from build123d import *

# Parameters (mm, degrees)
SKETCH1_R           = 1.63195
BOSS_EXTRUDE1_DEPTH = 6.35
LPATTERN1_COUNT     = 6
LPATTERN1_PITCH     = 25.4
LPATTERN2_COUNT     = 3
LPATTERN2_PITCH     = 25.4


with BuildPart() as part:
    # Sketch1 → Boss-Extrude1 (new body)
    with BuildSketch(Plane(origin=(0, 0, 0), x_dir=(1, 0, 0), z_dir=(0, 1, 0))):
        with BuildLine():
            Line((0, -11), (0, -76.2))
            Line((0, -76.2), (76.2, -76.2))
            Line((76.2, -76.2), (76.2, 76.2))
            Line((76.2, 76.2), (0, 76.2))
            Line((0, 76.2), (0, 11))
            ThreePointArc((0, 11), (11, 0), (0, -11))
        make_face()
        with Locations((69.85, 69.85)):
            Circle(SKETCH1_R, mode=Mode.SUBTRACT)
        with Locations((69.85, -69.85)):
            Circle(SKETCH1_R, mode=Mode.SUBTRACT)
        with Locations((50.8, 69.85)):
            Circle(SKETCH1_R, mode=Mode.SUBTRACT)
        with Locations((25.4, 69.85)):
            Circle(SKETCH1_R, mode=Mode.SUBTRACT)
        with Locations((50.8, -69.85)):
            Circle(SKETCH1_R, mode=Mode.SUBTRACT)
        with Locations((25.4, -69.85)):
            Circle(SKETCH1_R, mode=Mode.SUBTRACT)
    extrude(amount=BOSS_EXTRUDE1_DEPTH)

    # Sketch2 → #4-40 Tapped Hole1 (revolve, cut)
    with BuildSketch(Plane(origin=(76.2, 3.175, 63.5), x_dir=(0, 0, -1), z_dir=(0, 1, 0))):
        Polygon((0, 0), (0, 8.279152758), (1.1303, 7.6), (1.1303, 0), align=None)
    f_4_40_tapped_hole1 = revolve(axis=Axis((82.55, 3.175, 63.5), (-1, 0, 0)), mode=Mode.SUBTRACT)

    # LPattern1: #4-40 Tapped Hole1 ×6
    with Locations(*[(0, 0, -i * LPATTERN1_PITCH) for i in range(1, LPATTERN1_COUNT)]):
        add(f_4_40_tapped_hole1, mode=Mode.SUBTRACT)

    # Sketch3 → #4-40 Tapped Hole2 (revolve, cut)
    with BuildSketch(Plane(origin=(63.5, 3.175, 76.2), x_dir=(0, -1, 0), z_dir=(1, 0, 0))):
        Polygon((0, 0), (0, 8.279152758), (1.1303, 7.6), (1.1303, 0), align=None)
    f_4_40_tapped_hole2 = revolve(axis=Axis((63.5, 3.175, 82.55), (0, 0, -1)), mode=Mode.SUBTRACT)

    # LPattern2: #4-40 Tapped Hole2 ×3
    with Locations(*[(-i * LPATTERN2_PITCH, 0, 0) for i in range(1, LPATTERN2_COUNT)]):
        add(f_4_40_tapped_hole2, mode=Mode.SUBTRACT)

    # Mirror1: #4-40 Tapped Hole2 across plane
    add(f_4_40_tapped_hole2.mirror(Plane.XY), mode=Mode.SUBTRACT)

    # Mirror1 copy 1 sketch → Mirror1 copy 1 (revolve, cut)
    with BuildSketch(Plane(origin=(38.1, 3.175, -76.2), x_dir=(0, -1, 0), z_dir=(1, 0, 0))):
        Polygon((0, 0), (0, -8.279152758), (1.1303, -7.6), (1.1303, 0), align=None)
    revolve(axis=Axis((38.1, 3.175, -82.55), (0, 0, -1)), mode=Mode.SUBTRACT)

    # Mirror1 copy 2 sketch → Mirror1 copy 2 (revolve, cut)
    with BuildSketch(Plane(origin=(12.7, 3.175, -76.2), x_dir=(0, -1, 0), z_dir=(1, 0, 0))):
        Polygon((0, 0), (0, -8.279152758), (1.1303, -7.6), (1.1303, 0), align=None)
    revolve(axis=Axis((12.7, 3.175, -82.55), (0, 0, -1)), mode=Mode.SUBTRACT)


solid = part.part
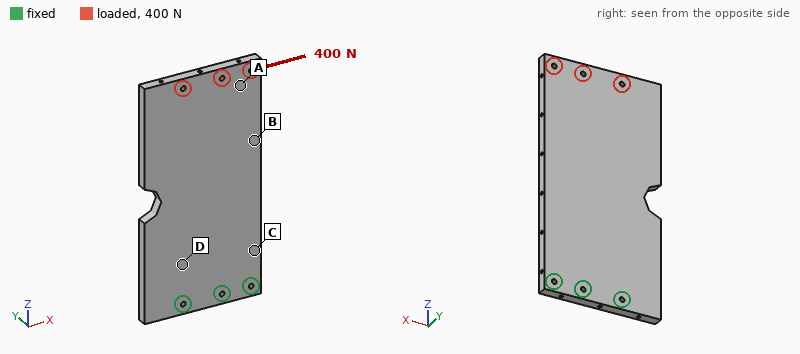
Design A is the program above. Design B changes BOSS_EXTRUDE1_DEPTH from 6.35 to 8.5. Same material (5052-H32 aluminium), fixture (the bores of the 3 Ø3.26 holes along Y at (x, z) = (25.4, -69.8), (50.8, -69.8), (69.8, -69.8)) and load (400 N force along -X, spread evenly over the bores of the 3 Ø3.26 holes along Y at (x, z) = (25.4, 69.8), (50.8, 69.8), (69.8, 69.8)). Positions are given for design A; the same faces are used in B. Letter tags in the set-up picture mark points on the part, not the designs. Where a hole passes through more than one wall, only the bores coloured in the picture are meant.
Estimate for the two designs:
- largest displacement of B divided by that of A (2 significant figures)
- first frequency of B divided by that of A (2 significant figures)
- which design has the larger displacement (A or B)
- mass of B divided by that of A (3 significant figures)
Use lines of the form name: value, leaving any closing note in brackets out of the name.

largest displacement of B divided by that of A: 0.74
first frequency of B divided by that of A: 1.3
which design has the larger displacement: A
mass of B divided by that of A: 1.34
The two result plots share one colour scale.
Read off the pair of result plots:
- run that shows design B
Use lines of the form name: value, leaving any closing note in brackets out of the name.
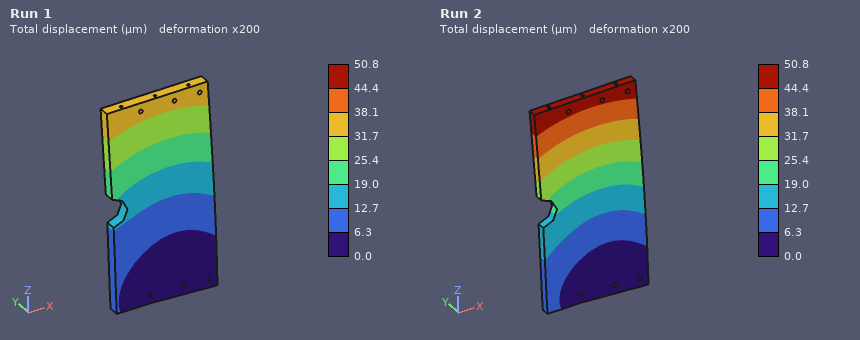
run that shows design B: Run 1
